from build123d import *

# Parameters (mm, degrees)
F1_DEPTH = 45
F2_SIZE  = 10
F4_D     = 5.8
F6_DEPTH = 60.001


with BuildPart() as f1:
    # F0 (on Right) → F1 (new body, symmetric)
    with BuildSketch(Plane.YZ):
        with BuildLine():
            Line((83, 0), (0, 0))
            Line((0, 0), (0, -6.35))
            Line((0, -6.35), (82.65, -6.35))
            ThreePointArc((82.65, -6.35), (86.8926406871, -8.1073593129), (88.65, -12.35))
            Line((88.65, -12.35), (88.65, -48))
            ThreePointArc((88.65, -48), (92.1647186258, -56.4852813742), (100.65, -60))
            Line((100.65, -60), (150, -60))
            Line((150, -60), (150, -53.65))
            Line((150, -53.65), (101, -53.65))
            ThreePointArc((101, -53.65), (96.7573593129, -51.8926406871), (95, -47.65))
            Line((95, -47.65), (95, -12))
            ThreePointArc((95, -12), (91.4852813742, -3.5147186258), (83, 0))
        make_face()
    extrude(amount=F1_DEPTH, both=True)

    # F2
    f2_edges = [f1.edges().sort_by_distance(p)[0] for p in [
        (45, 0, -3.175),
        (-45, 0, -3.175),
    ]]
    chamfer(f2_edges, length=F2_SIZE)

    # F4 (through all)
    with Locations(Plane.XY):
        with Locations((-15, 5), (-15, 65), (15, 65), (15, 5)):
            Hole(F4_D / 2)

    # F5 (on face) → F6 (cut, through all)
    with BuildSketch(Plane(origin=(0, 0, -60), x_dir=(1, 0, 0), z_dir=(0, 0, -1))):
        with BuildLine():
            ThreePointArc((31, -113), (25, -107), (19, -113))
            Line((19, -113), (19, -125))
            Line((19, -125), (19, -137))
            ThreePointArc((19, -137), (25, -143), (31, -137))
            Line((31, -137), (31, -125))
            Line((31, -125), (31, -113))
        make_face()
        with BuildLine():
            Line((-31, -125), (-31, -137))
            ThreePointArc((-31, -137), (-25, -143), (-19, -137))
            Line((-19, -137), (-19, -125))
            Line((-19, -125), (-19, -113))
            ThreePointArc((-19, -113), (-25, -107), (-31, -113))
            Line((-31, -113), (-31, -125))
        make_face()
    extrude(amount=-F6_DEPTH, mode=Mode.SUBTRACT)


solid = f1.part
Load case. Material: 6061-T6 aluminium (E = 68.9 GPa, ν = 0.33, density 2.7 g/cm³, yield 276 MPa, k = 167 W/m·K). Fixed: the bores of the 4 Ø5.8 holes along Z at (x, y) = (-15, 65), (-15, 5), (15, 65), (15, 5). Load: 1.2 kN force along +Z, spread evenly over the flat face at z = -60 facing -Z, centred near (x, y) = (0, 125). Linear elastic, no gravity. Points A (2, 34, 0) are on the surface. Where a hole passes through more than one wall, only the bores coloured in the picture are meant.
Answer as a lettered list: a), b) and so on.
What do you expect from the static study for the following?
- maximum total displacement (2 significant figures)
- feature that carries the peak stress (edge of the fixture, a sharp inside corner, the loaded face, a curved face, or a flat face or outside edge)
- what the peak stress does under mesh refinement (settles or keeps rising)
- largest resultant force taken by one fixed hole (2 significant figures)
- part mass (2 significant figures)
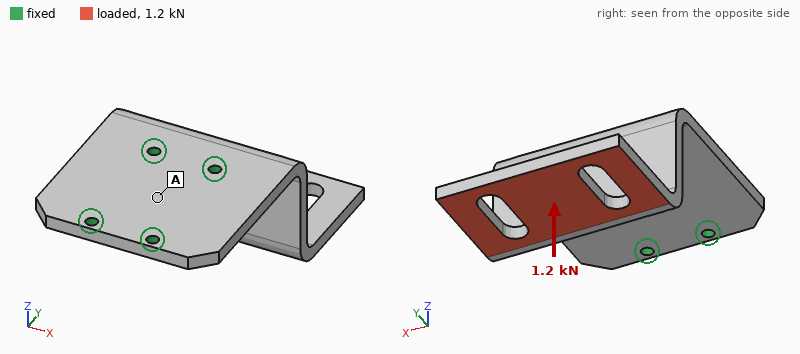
a) 2.2 mm
b) edge of the fixture
c) keeps rising
d) 770 N
e) 290 g
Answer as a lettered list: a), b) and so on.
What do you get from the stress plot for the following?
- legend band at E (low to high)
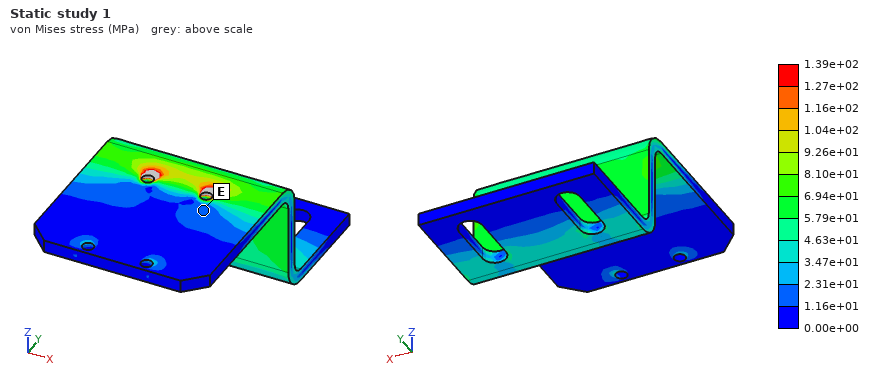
a) 1.16e+01 to 2.31e+01 MPa
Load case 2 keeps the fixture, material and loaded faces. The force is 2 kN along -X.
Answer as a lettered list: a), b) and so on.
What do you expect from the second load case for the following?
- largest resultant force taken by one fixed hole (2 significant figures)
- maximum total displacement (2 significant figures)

a) 3.6 kN
b) 0.73 mm
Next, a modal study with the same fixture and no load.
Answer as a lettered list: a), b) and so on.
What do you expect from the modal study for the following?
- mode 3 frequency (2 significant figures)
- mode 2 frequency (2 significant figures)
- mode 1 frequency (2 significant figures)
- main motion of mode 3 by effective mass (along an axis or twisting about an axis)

a) 1200 Hz
b) 1000 Hz
c) 420 Hz
d) along X
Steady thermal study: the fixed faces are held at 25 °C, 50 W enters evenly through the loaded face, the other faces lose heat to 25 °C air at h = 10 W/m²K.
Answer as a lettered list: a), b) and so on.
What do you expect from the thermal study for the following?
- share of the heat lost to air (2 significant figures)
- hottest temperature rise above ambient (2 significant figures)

a) 13 %
b) 56 K
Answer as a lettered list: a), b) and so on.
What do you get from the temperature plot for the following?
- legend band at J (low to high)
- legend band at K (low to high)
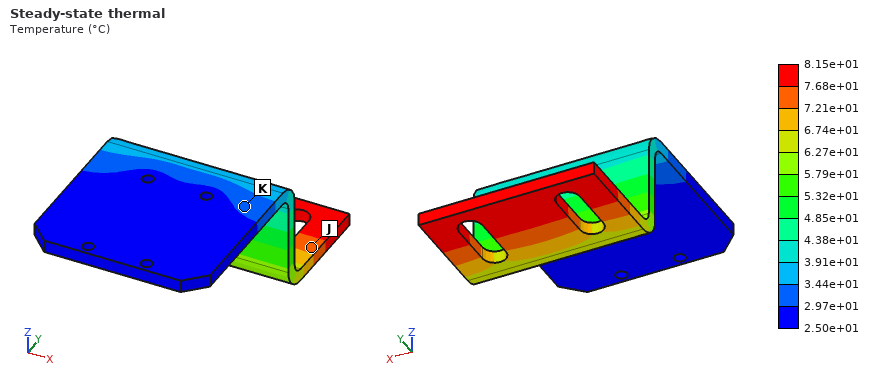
a) 7.21e+01 to 7.68e+01 °C
b) 2.97e+01 to 3.44e+01 °C
